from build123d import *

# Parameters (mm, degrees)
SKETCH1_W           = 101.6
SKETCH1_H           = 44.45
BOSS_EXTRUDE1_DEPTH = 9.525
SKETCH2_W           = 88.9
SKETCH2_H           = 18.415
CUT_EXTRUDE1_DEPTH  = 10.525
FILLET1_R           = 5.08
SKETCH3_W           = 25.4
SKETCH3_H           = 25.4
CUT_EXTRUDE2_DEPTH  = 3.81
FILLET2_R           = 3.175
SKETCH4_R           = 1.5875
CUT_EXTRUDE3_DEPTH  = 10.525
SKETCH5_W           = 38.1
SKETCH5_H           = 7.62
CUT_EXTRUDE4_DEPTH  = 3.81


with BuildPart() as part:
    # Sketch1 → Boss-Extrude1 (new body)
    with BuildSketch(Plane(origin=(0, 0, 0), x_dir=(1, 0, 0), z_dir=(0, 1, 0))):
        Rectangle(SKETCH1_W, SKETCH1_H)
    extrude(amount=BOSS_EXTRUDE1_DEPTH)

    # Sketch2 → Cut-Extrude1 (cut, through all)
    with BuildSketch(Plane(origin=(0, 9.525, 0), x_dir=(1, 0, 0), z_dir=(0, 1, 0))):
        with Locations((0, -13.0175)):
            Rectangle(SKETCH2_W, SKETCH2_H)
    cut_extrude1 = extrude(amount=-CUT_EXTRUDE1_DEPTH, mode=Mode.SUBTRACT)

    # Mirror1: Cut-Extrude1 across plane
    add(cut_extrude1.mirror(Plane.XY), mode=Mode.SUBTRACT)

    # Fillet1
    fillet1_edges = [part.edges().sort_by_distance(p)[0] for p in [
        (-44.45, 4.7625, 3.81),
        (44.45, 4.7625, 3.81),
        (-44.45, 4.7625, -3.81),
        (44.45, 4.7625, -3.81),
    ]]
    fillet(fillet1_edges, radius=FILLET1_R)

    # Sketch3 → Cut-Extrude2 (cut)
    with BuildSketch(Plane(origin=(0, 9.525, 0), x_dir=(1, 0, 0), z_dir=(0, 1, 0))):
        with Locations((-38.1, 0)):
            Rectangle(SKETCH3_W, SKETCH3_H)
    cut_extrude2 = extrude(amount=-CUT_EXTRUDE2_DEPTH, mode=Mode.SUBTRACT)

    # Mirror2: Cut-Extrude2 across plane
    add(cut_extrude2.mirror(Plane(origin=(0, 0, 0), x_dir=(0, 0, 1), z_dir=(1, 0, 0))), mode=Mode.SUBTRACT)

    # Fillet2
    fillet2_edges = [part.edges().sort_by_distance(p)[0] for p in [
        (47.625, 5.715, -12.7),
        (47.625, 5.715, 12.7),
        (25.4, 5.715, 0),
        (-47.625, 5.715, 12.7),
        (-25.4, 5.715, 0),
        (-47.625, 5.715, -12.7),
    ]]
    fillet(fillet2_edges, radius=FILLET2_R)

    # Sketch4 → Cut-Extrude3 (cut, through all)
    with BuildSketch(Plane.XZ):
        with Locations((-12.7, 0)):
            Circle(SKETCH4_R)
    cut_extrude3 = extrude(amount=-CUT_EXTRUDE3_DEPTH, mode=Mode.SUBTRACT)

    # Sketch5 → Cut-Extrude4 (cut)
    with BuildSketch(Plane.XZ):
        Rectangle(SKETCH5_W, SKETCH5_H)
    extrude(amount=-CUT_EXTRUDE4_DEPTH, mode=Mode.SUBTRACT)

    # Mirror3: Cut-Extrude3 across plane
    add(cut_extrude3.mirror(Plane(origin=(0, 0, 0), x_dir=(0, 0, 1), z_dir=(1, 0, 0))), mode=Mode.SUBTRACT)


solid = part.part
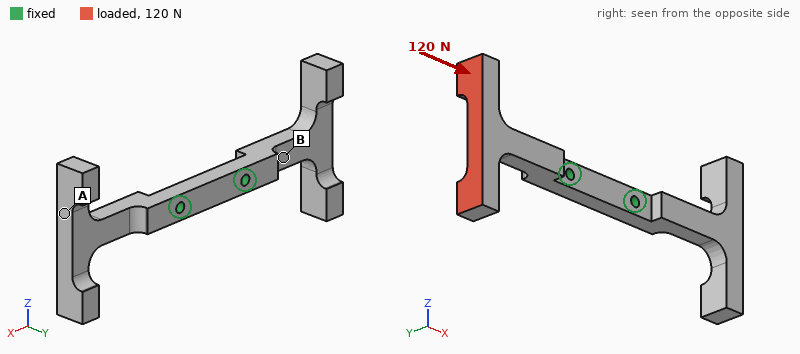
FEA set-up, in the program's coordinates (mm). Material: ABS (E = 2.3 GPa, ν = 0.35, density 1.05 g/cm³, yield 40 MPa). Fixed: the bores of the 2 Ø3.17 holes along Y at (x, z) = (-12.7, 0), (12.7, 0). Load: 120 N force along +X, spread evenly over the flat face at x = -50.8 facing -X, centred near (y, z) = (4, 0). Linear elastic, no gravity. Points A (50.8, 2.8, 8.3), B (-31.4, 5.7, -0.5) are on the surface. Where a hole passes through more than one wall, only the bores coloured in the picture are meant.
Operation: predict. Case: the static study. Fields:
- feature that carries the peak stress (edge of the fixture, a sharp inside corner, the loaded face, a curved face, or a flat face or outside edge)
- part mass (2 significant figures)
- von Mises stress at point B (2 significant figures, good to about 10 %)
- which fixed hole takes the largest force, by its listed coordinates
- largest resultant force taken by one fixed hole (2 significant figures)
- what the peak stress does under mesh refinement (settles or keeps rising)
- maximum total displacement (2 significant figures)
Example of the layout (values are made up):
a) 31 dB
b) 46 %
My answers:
a) edge of the fixture
b) 8.9 g
c) 6.0 MPa
d) (-12.7, 0)
e) 120 N
f) keeps rising
g) 0.34 mm
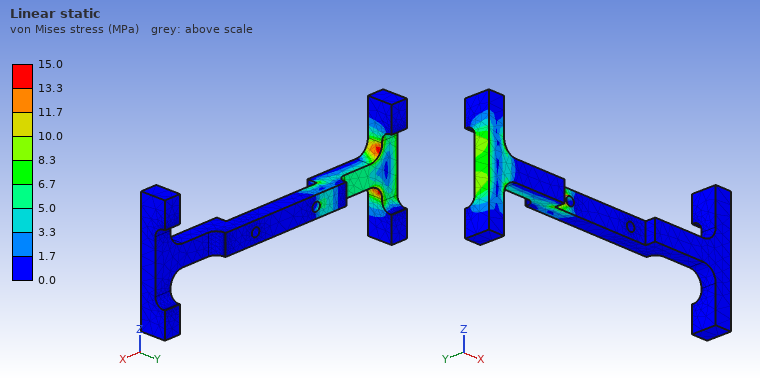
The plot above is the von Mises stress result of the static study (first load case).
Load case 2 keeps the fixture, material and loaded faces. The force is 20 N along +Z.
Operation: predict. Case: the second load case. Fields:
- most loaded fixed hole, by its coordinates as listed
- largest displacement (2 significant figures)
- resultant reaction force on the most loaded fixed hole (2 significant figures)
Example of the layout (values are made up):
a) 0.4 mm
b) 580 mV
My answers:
a) (-12.7, 0)
b) 1.1 mm
c) 28 N
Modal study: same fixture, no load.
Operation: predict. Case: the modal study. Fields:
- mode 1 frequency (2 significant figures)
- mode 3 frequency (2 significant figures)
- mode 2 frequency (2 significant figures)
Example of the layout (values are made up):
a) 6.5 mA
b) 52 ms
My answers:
a) 470 Hz
b) 480 Hz
c) 470 Hz
